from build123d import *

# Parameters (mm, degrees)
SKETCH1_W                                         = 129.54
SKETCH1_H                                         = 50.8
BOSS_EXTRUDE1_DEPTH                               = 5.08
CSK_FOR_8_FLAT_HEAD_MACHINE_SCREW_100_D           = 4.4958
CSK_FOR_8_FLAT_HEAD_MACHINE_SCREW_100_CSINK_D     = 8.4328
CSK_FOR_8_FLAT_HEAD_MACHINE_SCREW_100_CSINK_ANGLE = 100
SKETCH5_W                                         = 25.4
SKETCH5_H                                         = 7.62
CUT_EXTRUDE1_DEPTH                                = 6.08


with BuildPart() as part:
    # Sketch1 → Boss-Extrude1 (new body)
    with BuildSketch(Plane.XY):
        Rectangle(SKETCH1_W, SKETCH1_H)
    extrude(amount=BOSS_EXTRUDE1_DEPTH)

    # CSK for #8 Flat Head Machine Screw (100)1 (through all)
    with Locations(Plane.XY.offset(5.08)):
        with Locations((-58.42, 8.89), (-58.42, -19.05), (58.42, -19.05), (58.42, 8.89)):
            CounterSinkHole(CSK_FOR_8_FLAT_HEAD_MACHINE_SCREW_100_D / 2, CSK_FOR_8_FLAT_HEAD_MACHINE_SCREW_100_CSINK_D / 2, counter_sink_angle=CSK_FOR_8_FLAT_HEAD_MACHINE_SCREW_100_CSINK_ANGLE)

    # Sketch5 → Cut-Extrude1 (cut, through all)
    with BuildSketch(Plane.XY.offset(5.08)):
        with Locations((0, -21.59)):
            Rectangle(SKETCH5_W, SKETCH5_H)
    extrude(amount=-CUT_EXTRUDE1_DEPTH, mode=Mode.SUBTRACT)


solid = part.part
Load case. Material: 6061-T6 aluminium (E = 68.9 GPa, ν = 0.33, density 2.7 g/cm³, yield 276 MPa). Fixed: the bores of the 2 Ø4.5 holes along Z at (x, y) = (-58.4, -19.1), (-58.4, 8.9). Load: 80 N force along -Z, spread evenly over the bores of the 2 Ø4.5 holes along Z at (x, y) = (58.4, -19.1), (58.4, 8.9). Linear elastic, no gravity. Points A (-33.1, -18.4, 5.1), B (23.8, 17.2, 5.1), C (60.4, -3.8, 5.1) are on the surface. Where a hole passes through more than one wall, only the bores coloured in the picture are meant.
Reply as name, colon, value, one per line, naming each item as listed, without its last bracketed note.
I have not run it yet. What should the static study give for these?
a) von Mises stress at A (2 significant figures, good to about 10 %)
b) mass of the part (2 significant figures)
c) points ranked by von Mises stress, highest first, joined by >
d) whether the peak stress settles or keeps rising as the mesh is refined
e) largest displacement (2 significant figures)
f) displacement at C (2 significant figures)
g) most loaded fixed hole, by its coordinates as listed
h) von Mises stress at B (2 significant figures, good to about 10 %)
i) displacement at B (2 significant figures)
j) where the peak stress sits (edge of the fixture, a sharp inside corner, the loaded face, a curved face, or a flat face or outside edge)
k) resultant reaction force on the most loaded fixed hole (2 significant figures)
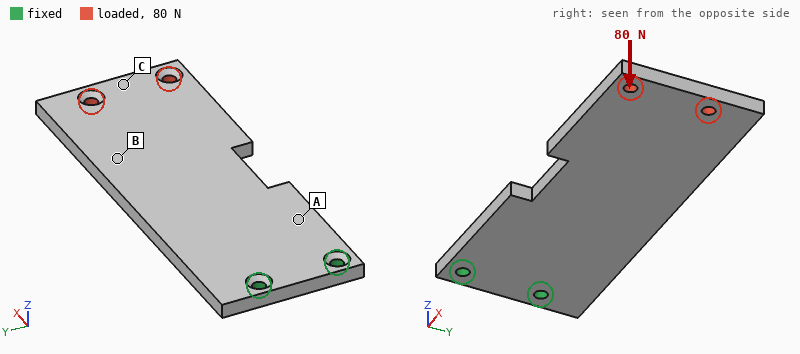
von Mises stress at A: 33 MPa
mass of the part: 86 g
points ranked by von Mises stress, highest first, joined by >: A > B > C
whether the peak stress settles or keeps rising as the mesh is refined: keeps rising
largest displacement: 1.4 mm
displacement at C: 1.3 mm
most loaded fixed hole, by its coordinates as listed: (-58.4, 8.9)
von Mises stress at B: 14 MPa
displacement at B: 0.73 mm
where the peak stress sits: edge of the fixture
resultant reaction force on the most loaded fixed hole: 63 N
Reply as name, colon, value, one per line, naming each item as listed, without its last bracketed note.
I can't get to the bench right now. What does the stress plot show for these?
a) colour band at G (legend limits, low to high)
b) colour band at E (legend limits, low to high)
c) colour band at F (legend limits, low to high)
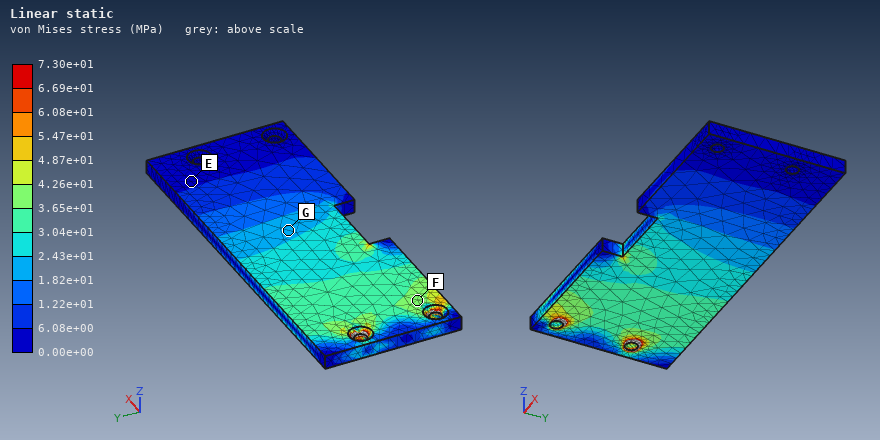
colour band at G: 1.82e+01 to 2.43e+01 MPa
colour band at E: 0.00e+00 to 6.08e+00 MPa
colour band at F: 3.65e+01 to 4.26e+01 MPa
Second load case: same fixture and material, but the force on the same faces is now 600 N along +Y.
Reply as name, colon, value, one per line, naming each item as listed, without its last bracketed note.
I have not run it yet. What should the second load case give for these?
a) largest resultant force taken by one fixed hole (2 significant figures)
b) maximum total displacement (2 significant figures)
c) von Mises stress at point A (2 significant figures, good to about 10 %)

largest resultant force taken by one fixed hole: 2.4 kN
maximum total displacement: 0.17 mm
von Mises stress at point A: 19 MPa
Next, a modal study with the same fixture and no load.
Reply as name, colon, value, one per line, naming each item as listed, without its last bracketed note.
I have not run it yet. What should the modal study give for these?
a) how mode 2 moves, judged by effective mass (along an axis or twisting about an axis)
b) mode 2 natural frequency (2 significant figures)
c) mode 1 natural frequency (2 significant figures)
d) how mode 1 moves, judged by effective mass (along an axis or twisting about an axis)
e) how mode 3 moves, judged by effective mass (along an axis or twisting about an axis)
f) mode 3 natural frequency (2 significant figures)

how mode 2 moves, judged by effective mass: twisting about X
mode 2 natural frequency: 1300 Hz
mode 1 natural frequency: 260 Hz
how mode 1 moves, judged by effective mass: along Z
how mode 3 moves, judged by effective mass: along Z
mode 3 natural frequency: 1600 Hz
